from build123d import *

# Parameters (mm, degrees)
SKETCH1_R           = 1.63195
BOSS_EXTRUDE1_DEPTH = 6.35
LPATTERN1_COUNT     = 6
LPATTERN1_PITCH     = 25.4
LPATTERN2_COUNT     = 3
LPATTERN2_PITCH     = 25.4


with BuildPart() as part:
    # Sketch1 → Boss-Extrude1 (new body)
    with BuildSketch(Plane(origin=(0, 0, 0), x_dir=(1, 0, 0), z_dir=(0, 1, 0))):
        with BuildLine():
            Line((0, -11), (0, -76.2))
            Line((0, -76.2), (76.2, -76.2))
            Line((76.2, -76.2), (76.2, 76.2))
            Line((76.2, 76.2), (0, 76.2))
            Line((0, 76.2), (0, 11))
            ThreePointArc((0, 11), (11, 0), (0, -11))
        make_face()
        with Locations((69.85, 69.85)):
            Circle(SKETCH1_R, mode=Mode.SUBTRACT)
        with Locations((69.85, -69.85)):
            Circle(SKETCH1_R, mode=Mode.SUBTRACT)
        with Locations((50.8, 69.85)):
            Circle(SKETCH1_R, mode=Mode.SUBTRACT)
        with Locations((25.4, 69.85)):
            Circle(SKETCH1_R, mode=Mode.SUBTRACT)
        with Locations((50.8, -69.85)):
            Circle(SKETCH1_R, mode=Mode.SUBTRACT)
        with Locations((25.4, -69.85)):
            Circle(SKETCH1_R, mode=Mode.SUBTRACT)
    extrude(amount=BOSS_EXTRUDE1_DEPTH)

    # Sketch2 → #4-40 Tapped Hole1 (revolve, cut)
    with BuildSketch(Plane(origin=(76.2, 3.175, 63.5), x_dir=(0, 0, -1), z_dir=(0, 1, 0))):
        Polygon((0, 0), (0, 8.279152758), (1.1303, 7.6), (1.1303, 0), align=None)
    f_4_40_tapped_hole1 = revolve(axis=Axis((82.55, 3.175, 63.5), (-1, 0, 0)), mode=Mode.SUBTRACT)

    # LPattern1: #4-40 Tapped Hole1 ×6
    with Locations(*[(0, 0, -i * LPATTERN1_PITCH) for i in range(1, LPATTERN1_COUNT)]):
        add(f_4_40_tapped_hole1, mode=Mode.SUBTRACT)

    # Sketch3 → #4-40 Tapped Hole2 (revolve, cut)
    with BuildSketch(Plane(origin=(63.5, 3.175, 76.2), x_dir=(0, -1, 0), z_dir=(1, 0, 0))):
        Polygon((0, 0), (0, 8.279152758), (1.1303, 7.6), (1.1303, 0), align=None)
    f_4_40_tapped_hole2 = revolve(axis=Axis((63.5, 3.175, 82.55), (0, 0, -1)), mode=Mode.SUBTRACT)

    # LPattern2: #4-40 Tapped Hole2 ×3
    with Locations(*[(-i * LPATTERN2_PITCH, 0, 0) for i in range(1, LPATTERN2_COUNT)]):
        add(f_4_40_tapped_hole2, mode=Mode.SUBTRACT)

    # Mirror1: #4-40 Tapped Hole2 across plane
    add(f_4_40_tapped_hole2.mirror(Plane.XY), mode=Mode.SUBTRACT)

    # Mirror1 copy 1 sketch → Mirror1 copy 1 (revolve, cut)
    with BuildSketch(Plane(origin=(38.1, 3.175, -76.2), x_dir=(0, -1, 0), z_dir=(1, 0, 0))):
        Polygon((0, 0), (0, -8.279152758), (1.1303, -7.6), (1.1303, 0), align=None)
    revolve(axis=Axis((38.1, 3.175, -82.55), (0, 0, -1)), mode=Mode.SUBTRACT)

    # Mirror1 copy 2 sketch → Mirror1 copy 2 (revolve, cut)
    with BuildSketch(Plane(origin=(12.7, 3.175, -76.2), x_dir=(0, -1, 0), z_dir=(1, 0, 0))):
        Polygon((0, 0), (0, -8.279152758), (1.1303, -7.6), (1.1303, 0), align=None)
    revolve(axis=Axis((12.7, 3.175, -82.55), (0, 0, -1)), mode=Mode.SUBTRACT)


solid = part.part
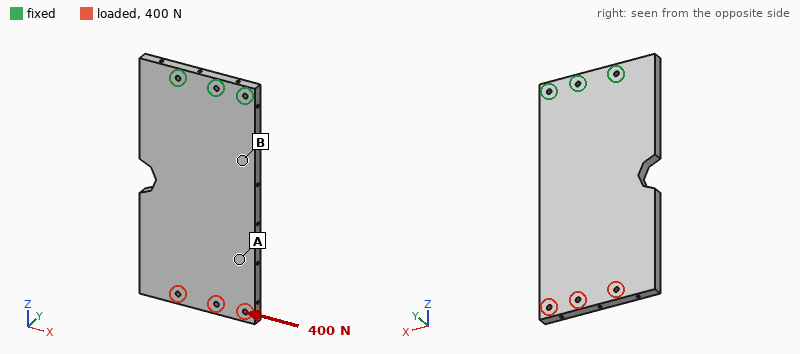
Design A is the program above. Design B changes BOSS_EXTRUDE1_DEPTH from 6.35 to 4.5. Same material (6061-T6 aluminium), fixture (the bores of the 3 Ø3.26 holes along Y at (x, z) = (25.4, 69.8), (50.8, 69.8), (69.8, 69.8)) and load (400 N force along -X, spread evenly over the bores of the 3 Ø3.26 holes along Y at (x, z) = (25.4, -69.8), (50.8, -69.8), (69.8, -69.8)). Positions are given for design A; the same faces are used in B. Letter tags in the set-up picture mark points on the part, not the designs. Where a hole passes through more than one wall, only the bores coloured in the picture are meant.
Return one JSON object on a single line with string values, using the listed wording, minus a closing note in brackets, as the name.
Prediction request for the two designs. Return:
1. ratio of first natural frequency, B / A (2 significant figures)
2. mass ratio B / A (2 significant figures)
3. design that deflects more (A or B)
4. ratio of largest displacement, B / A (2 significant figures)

{"ratio of first natural frequency, B / A": "0.72", "mass ratio B / A": "0.71", "design that deflects more": "B", "ratio of largest displacement, B / A": "1.5"}
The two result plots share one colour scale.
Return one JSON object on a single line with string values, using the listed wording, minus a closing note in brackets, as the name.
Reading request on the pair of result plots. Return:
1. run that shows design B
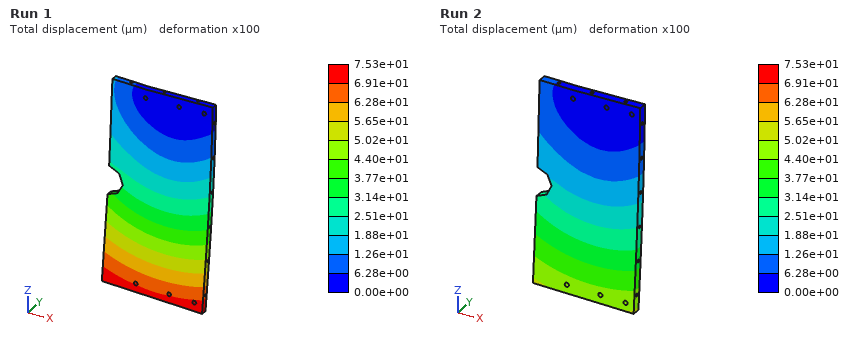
{"run that shows design B": "Run 1"}
